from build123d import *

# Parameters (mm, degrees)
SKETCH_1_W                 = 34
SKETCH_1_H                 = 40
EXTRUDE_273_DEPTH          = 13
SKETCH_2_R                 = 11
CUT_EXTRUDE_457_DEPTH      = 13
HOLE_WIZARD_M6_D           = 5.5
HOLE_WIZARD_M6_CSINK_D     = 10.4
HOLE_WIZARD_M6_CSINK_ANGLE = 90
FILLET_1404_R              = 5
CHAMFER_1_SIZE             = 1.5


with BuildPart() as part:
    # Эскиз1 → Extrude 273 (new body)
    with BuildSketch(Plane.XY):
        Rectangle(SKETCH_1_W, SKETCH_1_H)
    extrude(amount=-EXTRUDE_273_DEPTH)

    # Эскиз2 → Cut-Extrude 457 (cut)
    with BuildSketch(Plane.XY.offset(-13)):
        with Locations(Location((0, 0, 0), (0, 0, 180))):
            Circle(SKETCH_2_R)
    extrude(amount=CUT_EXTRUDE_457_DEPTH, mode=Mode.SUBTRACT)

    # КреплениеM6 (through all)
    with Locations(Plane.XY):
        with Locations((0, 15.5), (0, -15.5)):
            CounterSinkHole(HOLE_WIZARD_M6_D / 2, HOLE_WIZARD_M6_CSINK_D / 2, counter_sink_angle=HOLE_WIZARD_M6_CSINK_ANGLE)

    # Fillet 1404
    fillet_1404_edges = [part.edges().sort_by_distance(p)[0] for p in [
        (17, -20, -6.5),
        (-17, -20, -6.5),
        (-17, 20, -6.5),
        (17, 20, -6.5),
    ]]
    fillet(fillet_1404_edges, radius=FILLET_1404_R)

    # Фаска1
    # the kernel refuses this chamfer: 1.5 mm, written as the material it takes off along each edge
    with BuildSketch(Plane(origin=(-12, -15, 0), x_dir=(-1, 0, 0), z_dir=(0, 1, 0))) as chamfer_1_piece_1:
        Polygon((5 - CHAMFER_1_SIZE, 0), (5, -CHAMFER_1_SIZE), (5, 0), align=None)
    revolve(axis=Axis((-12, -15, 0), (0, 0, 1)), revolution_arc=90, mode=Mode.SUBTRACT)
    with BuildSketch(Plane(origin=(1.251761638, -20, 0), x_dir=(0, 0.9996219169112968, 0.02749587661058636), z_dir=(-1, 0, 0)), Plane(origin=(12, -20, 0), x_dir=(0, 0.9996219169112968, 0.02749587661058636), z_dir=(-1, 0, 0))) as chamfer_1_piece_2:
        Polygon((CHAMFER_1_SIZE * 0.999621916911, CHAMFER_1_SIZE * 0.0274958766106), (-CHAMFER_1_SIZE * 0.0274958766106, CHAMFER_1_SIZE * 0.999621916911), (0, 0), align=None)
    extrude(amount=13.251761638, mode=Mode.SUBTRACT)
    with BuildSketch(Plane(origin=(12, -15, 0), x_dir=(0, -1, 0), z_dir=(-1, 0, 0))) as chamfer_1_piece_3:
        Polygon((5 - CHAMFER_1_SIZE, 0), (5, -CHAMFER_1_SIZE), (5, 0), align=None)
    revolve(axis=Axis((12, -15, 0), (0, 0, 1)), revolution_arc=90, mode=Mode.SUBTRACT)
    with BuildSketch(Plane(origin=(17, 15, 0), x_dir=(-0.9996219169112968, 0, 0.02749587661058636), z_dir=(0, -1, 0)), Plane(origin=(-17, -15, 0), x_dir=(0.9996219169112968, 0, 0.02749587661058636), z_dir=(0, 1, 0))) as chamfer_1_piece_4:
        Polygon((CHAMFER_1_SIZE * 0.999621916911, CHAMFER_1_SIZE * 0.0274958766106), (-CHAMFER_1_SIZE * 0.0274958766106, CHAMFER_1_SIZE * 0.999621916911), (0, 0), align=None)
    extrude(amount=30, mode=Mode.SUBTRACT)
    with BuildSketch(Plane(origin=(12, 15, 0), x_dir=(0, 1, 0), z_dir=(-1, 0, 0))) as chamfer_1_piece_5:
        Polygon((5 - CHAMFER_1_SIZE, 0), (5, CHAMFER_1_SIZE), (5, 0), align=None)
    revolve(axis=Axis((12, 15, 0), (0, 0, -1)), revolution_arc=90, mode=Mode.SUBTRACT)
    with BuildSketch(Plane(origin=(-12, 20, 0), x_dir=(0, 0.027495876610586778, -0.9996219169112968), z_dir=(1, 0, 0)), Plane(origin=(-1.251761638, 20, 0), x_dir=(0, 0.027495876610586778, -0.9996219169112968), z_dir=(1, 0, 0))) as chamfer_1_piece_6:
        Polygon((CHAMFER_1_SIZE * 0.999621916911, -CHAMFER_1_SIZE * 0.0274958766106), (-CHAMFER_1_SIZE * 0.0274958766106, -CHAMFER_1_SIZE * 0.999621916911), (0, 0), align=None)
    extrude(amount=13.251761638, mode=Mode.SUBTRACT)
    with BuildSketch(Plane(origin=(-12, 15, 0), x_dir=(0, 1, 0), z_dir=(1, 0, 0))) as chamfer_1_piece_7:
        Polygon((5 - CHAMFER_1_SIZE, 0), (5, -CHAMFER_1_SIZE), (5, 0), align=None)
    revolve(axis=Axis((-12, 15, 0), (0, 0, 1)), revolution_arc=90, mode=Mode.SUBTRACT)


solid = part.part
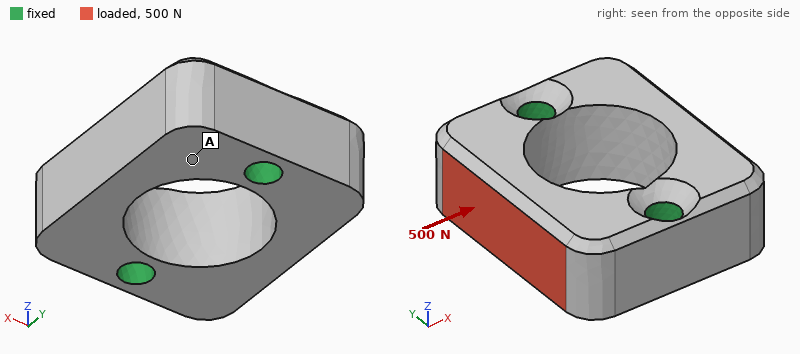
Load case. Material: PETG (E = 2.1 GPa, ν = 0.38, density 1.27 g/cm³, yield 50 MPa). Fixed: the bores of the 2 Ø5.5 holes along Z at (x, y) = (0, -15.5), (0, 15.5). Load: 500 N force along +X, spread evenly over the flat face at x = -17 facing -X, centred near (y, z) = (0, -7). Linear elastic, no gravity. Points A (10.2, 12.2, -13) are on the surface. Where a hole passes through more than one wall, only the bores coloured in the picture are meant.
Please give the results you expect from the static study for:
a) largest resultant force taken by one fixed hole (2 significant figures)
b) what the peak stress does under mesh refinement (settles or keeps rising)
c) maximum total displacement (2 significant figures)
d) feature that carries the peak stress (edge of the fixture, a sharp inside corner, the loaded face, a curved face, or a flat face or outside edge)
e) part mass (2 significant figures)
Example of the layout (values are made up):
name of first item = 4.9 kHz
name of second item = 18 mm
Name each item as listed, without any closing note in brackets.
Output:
largest resultant force taken by one fixed hole = 280 N
what the peak stress does under mesh refinement = keeps rising
maximum total displacement = 46 µm
feature that carries the peak stress = edge of the fixture
part mass = 15 g
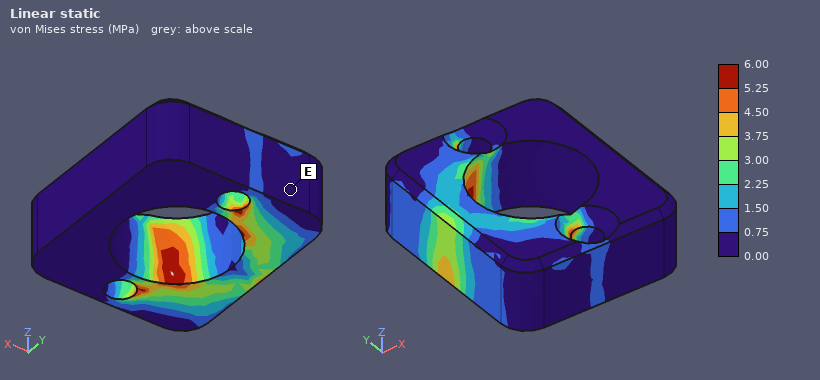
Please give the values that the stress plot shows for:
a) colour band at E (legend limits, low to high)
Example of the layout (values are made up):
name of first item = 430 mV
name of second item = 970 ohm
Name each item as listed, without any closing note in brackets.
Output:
colour band at E = 0.00 to 0.75 MPa
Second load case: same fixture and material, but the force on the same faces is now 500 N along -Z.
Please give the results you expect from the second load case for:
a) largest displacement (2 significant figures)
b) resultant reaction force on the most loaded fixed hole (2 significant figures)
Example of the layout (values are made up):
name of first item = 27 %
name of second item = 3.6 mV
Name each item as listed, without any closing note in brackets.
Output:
largest displacement = 0.23 mm
resultant reaction force on the most loaded fixed hole = 250 N
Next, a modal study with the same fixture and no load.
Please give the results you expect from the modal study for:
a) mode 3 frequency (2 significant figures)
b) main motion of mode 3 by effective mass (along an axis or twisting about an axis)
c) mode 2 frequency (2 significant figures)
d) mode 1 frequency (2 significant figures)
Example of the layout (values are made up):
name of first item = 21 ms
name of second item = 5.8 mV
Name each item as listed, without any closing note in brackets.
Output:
mode 3 frequency = 6400 Hz
main motion of mode 3 by effective mass = twisting about Z
mode 2 frequency = 5100 Hz
mode 1 frequency = 4900 Hz
